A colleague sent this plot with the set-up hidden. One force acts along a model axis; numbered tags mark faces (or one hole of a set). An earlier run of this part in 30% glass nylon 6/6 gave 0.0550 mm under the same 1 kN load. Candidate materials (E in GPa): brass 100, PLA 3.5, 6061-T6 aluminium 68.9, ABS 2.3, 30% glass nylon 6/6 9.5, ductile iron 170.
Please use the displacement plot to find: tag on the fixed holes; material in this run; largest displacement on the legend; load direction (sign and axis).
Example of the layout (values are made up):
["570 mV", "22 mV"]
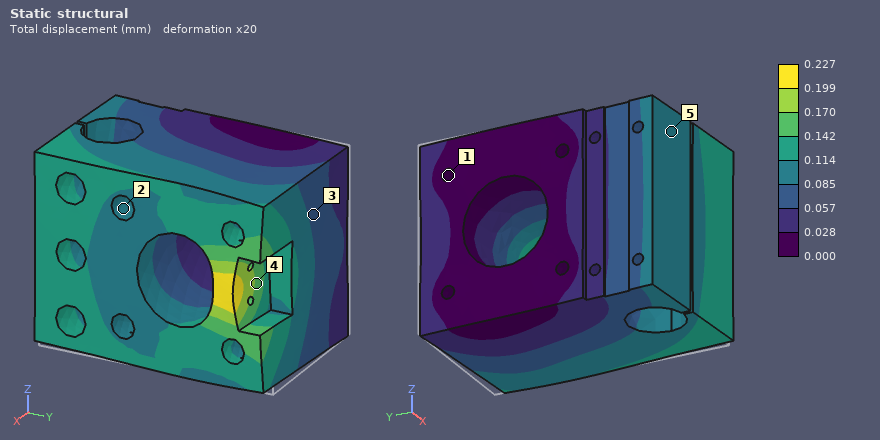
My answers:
["1", "ABS", "0.227 mm", "-Y"]
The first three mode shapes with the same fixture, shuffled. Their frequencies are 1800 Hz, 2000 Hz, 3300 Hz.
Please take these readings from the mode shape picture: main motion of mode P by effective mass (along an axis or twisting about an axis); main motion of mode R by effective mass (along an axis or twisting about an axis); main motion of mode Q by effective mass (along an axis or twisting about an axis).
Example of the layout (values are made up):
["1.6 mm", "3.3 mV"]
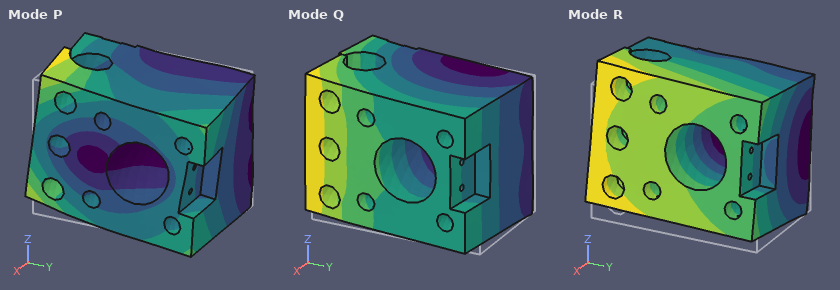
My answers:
["twisting about X", "along Z", "along Y"]
